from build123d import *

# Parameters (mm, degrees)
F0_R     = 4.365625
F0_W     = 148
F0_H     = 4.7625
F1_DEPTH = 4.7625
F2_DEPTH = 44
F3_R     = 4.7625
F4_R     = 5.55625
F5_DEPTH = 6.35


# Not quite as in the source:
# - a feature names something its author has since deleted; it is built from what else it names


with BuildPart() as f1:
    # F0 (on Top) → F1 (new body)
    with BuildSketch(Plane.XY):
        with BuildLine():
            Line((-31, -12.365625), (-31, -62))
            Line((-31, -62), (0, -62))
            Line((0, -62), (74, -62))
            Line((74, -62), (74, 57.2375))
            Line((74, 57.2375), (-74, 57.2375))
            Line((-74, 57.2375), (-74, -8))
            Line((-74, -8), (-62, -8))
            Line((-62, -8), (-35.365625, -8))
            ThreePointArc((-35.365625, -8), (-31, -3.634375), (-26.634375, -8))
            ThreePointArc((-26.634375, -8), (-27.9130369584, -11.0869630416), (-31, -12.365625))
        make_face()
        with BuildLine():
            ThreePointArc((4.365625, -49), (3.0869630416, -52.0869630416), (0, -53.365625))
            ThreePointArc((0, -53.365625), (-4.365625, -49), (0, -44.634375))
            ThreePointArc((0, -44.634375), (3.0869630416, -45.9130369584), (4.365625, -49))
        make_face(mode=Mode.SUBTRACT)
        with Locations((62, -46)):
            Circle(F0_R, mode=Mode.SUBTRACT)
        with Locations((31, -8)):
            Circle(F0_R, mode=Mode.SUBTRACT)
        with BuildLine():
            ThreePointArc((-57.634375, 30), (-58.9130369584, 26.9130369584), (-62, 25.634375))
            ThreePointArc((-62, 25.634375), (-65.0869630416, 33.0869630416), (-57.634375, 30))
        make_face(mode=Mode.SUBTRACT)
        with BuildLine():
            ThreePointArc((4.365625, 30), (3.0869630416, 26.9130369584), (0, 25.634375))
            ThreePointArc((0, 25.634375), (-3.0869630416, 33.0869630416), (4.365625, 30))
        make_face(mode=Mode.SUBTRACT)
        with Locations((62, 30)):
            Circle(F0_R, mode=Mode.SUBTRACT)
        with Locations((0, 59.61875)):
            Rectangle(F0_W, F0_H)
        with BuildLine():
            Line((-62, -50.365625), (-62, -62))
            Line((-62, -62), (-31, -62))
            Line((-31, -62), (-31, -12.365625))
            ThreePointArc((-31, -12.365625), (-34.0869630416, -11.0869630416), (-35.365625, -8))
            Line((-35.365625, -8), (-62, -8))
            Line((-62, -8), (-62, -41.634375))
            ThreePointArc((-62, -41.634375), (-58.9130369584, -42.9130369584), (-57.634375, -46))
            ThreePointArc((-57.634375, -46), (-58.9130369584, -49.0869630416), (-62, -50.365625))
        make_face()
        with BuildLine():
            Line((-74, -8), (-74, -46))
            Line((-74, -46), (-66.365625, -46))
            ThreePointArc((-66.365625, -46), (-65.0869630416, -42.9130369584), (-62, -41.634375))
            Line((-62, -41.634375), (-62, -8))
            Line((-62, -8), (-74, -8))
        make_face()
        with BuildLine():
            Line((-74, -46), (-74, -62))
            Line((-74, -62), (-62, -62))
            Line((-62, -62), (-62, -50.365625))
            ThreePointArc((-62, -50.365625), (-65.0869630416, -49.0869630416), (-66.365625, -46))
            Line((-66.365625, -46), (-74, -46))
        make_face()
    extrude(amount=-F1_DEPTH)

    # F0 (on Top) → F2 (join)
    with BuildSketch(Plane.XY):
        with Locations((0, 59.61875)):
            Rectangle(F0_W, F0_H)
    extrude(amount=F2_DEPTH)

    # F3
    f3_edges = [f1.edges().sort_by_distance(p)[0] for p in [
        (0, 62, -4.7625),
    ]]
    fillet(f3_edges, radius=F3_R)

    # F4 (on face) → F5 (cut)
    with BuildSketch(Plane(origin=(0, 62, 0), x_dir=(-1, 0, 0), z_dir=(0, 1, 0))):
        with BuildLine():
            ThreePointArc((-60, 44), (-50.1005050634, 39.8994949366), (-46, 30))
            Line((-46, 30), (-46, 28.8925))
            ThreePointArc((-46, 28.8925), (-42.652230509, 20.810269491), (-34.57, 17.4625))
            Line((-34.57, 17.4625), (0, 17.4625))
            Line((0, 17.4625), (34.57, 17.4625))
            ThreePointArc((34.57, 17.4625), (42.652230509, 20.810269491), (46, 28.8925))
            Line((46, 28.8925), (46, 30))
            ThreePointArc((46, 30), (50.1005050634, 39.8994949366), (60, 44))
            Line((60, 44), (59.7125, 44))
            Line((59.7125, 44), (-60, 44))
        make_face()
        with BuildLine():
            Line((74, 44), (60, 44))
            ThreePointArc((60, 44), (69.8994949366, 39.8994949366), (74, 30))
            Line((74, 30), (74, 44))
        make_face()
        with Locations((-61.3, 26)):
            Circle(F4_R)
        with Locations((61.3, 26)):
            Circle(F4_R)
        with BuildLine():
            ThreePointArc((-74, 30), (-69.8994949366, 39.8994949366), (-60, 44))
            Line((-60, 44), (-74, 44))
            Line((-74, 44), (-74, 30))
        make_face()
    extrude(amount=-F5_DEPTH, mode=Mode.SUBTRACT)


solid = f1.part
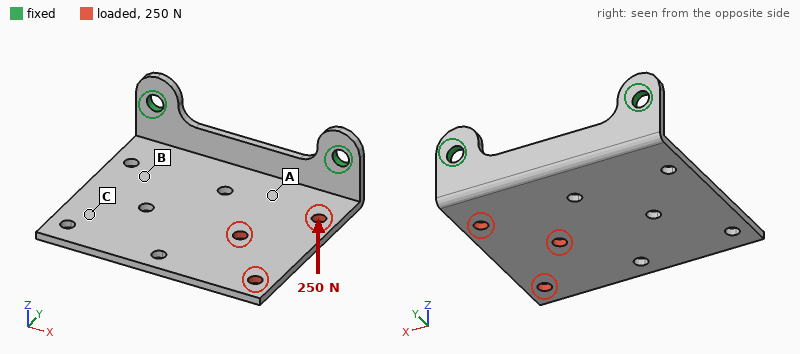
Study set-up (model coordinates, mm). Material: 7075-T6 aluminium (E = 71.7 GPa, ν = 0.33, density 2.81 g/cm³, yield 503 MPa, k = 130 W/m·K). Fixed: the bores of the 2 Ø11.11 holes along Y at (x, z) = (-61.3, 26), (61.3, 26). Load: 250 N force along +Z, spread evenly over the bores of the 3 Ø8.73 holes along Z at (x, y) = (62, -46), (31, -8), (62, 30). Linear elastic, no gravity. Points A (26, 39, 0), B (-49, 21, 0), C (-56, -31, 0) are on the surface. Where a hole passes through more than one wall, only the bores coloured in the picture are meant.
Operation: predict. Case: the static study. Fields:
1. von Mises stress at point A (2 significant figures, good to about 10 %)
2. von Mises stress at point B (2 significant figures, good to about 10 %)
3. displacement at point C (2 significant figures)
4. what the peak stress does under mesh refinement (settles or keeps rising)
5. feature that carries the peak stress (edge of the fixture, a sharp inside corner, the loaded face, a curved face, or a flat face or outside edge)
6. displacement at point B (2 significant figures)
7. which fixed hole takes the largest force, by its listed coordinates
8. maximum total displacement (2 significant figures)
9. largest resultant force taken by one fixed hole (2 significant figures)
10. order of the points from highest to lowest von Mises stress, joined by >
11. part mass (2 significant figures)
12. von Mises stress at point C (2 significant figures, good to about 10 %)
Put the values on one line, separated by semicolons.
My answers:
24 MPa; 16 MPa; 0.94 mm; keeps rising; edge of the fixture; 0.34 mm; (61.3, 26); 2.0 mm; 240 N; A > B > C; 290 g; 6.5 MPa
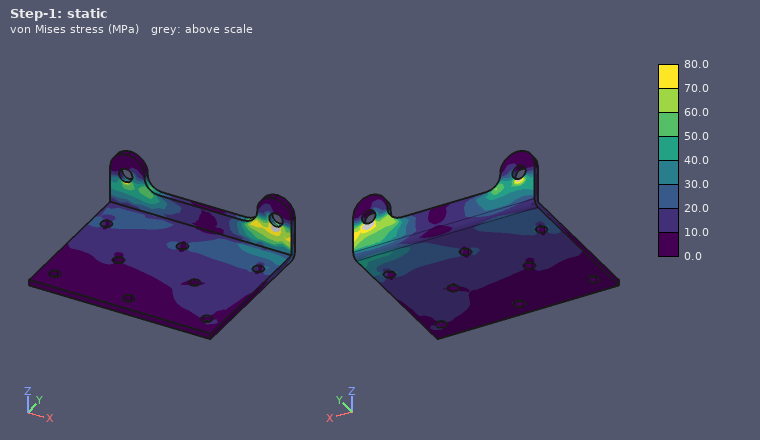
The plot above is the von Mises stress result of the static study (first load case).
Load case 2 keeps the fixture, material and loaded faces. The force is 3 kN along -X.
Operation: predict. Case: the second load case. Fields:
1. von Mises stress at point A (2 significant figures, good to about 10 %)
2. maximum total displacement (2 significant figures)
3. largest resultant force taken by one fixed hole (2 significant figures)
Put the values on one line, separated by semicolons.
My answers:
36 MPa; 0.84 mm; 2.3 kN
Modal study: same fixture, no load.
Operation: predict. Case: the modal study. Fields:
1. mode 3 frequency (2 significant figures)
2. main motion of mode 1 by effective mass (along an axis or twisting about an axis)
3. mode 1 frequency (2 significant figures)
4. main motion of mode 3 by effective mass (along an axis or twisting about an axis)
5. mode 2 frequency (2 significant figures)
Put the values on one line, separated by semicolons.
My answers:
930 Hz; along Z; 170 Hz; along X; 480 Hz
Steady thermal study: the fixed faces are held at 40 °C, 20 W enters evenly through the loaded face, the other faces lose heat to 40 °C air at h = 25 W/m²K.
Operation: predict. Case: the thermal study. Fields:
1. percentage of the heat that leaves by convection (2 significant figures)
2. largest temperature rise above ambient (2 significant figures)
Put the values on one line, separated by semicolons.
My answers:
55 %; 23 K
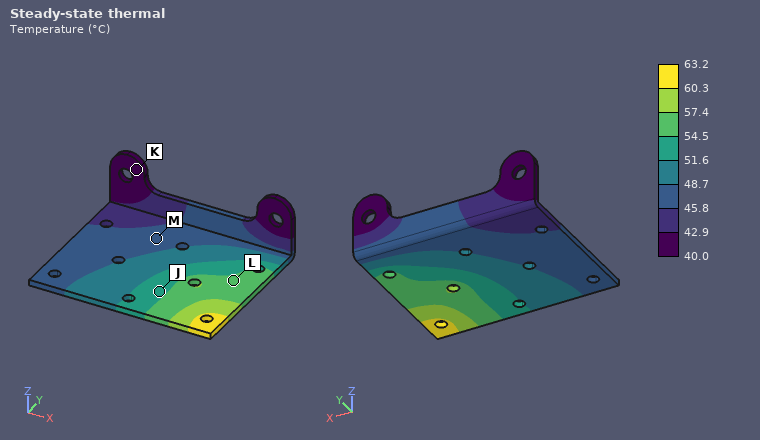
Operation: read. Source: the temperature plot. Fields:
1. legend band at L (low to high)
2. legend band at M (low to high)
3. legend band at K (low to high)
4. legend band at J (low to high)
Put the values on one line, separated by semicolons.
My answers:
54.5 to 57.4 °C; 45.8 to 48.7 °C; 40.0 to 42.9 °C; 51.6 to 54.5 °C
